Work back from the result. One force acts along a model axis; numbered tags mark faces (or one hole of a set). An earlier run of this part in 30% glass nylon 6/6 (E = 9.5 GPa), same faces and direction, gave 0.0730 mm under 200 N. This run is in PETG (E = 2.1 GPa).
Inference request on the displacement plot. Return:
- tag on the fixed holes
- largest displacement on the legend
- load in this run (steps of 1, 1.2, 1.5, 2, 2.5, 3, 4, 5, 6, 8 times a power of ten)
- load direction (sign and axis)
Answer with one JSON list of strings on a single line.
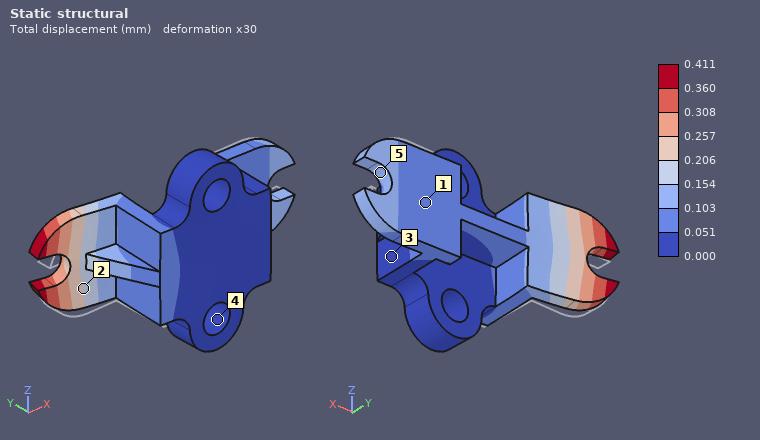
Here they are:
["4", "0.411 mm", "250 N", "+Y"]
